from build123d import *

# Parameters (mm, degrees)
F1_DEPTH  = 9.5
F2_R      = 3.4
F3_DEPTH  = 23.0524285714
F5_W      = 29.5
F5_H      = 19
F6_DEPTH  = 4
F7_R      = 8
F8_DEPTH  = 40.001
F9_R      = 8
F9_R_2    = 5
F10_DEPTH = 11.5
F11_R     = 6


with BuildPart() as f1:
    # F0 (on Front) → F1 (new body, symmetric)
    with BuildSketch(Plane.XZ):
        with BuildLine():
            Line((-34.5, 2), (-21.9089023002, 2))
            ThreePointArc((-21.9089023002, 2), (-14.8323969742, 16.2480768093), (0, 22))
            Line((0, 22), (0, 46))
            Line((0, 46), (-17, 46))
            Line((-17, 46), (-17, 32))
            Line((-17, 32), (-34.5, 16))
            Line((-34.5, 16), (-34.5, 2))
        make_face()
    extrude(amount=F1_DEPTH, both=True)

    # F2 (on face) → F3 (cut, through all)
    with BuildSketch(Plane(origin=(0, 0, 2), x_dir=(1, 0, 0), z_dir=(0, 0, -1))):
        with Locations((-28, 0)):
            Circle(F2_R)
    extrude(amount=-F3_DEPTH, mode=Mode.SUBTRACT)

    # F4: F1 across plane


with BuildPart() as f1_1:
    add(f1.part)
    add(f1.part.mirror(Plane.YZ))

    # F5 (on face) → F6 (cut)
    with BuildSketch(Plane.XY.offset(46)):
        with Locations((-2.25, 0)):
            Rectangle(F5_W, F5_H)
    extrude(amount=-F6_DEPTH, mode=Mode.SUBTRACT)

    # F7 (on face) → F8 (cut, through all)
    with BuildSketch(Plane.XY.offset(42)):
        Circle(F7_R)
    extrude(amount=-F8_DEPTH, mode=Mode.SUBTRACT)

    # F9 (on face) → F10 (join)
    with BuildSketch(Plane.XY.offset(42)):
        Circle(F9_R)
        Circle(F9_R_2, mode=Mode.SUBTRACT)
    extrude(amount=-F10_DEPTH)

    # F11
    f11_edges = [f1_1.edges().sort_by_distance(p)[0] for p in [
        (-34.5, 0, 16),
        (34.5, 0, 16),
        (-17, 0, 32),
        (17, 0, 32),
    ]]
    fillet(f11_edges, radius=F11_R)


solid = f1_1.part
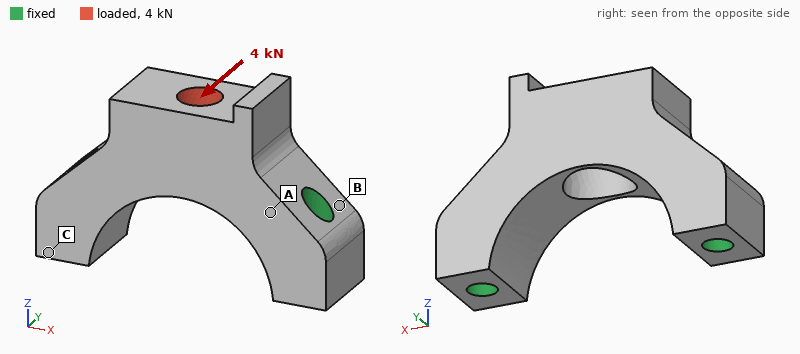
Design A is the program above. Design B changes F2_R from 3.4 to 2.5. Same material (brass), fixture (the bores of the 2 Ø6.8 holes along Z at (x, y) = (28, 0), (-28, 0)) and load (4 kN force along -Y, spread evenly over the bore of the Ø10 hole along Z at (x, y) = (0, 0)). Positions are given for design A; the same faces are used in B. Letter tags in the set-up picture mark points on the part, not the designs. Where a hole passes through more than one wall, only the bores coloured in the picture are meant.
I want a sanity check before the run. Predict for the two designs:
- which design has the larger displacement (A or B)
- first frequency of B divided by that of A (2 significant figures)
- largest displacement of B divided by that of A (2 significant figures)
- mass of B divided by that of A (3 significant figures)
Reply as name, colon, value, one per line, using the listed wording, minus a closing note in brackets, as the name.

which design has the larger displacement: B
first frequency of B divided by that of A: 0.90
largest displacement of B divided by that of A: 1.2
mass of B divided by that of A: 1.03
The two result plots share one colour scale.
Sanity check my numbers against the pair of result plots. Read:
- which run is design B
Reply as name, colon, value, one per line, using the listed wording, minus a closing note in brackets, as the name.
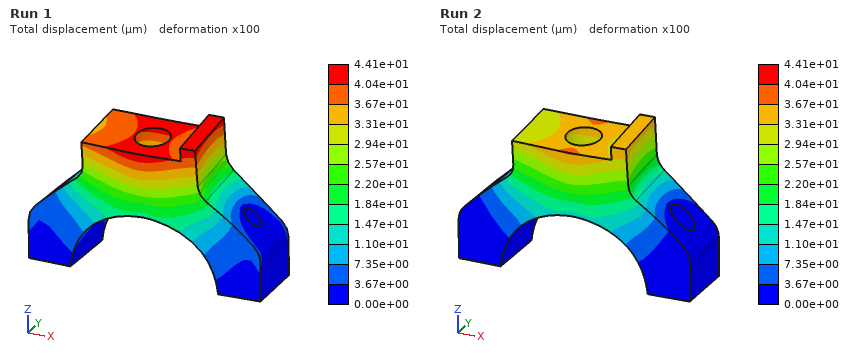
which run is design B: Run 1
